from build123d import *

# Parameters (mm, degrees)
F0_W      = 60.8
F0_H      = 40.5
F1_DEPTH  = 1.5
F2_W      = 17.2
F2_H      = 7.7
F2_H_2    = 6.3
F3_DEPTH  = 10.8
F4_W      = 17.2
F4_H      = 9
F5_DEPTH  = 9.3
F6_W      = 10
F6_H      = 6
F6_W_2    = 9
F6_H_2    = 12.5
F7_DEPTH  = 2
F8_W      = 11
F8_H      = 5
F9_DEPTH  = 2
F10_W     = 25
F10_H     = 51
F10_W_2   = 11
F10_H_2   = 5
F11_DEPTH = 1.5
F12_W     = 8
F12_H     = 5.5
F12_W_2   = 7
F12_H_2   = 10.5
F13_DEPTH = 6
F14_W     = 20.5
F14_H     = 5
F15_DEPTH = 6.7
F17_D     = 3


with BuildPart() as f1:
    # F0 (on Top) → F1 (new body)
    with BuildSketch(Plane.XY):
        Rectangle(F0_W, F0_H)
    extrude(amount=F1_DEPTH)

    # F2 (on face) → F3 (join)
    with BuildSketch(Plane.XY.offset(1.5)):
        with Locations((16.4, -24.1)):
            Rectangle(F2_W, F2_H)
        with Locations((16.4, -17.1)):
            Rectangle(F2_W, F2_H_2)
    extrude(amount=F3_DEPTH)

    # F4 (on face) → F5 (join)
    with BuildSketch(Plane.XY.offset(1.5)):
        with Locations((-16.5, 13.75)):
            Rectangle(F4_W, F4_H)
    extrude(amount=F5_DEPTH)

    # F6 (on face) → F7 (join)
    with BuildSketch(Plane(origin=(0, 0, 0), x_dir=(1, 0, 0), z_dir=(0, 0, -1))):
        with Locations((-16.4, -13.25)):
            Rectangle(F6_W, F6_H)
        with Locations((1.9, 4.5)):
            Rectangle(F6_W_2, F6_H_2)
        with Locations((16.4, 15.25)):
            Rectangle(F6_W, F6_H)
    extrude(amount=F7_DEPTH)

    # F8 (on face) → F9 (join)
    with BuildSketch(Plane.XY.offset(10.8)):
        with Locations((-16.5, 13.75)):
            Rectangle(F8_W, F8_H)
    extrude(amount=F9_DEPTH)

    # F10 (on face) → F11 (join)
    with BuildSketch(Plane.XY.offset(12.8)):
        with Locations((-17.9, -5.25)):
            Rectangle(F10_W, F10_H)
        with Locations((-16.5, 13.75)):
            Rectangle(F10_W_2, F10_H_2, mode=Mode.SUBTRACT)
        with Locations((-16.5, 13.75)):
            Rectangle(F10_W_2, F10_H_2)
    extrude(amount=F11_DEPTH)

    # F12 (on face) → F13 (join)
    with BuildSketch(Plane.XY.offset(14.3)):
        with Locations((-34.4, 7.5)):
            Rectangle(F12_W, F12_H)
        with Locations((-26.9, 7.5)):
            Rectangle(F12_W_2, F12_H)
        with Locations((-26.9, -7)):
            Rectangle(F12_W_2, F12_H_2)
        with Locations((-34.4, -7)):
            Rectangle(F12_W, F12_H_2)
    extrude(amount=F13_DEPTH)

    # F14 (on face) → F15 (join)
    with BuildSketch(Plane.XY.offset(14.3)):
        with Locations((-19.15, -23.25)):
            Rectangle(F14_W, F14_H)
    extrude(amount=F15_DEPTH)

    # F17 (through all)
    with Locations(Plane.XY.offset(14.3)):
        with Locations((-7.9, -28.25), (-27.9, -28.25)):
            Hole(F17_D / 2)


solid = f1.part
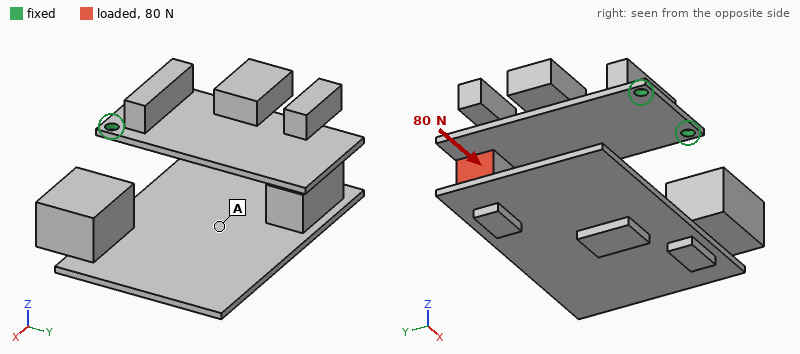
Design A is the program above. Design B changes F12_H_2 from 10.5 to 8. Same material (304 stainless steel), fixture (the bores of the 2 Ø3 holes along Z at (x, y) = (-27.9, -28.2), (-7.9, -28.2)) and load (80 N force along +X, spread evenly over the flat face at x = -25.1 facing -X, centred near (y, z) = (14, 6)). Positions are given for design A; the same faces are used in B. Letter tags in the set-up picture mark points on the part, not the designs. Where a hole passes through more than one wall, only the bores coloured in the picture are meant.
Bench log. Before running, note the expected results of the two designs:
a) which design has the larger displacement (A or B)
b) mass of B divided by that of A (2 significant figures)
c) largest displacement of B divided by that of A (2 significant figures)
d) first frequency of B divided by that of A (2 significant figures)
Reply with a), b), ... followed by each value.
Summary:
a) B
b) 0.98
c) 1.1
d) 0.98
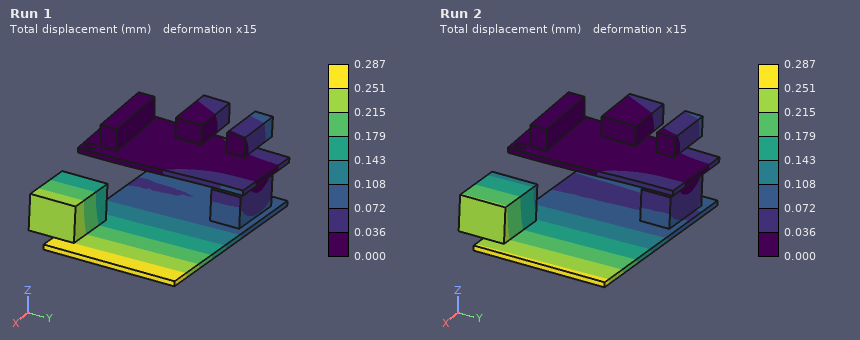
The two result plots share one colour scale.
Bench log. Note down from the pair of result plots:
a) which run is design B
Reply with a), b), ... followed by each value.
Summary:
a) Run 1
